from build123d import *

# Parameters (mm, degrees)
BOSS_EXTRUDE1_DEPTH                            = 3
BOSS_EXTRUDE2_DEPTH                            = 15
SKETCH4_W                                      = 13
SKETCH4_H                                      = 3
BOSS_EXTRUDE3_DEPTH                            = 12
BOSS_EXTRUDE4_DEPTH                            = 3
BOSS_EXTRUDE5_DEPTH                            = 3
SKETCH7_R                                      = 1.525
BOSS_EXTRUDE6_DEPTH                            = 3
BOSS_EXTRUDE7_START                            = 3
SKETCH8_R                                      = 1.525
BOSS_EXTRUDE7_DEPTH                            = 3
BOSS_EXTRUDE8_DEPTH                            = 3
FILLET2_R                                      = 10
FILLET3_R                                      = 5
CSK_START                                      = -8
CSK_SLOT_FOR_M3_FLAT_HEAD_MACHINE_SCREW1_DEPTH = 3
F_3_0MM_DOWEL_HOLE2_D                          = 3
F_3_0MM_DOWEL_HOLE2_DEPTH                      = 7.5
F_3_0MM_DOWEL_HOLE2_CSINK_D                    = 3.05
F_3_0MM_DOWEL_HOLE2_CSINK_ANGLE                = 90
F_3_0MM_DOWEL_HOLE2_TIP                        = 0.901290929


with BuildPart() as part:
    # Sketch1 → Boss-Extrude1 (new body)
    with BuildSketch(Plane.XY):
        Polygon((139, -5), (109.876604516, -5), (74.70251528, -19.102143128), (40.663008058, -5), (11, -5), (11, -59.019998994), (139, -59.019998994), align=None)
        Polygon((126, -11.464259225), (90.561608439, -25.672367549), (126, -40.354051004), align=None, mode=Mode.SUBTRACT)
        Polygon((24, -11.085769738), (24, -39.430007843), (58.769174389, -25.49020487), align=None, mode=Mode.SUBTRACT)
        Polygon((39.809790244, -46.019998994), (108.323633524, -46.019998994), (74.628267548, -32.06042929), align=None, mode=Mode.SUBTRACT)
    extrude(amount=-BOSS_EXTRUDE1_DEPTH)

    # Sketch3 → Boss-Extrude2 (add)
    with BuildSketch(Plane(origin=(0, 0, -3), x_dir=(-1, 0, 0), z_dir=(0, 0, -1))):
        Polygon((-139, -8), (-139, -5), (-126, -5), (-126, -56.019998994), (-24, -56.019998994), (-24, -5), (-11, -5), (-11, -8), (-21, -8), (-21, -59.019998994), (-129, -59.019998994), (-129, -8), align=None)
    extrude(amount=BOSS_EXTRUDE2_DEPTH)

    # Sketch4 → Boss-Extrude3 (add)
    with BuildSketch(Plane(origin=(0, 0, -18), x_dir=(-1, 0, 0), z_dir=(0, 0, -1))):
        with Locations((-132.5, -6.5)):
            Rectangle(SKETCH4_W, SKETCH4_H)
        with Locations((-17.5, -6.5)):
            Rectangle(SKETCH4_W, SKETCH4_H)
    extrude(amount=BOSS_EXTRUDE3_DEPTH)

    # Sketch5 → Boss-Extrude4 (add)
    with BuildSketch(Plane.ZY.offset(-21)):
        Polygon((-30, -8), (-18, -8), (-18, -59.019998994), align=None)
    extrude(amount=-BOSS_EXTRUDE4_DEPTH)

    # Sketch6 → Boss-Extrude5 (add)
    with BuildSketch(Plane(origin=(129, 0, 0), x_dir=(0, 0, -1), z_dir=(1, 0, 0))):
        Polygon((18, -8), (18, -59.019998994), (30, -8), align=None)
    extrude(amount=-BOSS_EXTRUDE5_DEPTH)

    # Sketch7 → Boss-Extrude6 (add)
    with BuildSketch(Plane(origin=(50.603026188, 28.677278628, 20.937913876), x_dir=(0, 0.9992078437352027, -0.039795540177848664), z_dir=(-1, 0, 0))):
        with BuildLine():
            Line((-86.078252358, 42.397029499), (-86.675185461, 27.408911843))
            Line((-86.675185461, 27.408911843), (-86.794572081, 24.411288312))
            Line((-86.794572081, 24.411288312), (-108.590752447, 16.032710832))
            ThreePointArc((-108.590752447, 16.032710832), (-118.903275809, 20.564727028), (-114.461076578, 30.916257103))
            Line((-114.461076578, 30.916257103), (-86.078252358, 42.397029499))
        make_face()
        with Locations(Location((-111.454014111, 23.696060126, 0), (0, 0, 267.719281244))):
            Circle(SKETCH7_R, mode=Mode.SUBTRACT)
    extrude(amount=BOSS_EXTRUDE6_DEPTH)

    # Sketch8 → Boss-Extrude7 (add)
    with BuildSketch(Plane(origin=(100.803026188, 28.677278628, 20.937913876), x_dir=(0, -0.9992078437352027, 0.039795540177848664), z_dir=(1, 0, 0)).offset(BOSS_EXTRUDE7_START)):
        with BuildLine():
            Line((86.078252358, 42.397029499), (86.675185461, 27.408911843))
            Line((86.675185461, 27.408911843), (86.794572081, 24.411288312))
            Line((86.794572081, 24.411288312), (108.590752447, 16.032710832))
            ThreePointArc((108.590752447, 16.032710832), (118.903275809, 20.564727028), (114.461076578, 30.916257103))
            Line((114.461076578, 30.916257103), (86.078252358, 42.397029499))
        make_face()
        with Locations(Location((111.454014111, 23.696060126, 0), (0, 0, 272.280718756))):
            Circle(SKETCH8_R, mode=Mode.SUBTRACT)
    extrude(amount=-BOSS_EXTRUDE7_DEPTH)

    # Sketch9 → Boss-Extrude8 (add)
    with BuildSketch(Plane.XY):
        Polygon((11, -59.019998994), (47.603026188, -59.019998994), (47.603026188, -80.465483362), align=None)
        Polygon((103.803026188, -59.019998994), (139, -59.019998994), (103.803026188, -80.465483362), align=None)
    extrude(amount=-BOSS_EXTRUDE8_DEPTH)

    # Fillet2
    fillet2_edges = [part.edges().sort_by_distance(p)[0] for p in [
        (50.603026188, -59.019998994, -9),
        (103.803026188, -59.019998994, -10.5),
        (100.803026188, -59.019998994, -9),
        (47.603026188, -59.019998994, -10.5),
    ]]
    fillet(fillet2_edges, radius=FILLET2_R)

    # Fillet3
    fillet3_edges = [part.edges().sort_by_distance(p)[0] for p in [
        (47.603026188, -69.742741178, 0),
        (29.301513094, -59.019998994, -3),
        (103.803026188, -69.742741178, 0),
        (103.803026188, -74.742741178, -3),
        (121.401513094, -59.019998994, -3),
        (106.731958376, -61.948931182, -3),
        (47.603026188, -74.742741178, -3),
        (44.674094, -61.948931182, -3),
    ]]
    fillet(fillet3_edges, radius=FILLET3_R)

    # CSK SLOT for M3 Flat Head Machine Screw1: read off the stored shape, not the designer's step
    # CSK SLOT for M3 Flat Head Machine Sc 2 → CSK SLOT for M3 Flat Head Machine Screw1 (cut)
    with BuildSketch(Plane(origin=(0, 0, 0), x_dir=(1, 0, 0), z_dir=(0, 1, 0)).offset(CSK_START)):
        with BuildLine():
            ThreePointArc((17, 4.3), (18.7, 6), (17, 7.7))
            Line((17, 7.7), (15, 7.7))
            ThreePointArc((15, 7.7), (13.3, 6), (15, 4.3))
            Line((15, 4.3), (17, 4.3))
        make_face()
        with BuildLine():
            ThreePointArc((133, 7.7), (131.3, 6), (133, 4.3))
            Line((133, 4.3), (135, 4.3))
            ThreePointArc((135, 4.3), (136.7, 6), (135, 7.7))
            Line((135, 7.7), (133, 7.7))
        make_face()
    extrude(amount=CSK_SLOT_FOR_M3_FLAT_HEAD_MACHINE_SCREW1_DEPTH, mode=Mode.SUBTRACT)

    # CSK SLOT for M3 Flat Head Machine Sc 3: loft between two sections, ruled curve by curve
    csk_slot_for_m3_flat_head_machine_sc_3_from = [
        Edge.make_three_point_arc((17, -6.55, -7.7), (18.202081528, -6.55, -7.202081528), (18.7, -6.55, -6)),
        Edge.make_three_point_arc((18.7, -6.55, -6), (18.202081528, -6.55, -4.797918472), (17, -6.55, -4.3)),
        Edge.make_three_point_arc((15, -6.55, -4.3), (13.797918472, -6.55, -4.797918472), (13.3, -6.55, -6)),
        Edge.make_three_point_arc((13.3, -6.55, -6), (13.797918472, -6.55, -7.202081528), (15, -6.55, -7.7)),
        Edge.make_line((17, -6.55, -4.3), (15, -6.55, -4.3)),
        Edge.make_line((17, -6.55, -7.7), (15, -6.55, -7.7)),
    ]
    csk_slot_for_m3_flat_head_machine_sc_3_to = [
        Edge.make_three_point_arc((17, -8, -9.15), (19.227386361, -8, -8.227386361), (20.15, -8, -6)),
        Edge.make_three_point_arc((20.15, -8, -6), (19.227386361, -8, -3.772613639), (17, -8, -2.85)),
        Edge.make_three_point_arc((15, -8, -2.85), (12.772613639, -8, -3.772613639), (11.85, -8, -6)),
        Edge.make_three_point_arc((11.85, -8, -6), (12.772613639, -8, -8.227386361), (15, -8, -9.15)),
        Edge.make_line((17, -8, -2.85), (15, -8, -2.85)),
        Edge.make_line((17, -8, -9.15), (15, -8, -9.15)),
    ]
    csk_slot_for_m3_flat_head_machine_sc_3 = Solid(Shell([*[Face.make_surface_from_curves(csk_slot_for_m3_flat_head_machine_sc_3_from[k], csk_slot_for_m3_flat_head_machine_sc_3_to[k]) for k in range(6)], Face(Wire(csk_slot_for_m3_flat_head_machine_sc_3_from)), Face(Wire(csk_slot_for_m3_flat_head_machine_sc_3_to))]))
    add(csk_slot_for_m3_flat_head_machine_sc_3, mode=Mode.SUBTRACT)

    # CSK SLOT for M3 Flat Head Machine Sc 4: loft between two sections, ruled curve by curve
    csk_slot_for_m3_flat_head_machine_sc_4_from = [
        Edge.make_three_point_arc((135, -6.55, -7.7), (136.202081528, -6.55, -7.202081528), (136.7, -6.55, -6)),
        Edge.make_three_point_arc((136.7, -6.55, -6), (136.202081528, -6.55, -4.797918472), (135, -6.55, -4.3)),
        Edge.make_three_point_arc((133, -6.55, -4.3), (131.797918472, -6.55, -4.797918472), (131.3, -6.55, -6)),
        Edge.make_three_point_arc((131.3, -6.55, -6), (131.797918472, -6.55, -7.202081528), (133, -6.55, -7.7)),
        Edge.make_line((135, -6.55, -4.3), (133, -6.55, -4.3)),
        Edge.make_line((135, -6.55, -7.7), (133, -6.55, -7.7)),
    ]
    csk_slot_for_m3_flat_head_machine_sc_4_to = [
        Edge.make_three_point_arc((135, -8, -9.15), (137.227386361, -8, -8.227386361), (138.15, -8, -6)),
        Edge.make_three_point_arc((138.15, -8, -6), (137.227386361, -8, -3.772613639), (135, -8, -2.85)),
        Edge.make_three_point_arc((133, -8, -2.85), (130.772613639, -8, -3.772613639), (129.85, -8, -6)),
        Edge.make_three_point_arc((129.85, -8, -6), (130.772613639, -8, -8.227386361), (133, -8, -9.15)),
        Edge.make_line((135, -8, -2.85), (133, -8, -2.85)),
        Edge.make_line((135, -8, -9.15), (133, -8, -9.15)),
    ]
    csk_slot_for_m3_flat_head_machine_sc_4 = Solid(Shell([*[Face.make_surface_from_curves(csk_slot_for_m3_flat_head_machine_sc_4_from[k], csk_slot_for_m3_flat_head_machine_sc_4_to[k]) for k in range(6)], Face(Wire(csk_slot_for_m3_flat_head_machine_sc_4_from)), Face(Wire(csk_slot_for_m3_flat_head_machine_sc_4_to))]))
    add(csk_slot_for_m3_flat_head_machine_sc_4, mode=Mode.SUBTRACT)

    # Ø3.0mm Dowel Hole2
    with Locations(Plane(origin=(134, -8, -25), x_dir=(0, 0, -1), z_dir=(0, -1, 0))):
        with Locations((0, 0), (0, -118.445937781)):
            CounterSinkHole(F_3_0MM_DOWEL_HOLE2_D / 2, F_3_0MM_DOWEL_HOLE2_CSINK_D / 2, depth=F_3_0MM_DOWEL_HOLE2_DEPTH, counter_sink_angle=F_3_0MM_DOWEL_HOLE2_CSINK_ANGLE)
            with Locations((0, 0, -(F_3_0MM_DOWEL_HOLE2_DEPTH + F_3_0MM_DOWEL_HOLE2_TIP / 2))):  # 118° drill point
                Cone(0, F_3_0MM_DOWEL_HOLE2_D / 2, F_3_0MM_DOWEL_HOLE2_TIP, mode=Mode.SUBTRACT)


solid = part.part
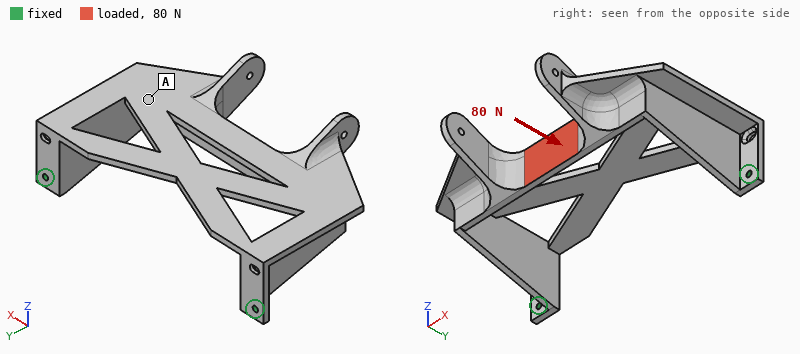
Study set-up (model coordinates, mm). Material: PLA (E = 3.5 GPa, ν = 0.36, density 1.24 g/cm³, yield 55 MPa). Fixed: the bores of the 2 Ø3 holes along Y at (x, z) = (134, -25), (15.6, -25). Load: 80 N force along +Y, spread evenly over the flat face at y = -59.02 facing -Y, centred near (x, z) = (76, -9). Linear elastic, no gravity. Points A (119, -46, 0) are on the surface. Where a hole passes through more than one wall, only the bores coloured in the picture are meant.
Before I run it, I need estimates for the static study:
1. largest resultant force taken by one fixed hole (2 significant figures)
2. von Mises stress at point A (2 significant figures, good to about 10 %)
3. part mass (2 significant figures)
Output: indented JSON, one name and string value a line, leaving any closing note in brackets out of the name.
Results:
{
  "largest resultant force taken by one fixed hole": "41 N",
  "von Mises stress at point A": "2.3 MPa",
  "part mass": "44 g"
}
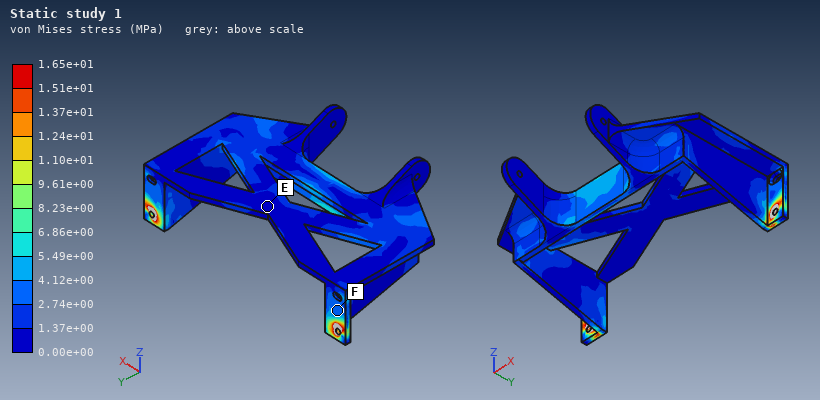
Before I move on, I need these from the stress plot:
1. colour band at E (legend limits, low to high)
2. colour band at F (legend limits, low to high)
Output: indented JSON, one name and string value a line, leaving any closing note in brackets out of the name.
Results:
{
  "colour band at E": "0.00e+00 to 1.37e+00 MPa",
  "colour band at F": "2.74e+00 to 4.12e+00 MPa"
}
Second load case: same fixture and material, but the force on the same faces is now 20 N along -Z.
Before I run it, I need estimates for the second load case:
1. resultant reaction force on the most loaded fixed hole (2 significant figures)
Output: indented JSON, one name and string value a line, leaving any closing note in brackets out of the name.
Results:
{
  "resultant reaction force on the most loaded fixed hole": "10 N"
}
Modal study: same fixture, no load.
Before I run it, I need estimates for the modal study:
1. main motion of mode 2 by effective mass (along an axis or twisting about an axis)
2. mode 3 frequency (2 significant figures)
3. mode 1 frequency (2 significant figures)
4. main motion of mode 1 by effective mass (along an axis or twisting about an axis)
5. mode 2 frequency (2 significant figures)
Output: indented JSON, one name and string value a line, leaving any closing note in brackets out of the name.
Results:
{
  "main motion of mode 2 by effective mass": "along X",
  "mode 3 frequency": "500 Hz",
  "mode 1 frequency": "130 Hz",
  "main motion of mode 1 by effective mass": "along Z",
  "mode 2 frequency": "230 Hz"
}
